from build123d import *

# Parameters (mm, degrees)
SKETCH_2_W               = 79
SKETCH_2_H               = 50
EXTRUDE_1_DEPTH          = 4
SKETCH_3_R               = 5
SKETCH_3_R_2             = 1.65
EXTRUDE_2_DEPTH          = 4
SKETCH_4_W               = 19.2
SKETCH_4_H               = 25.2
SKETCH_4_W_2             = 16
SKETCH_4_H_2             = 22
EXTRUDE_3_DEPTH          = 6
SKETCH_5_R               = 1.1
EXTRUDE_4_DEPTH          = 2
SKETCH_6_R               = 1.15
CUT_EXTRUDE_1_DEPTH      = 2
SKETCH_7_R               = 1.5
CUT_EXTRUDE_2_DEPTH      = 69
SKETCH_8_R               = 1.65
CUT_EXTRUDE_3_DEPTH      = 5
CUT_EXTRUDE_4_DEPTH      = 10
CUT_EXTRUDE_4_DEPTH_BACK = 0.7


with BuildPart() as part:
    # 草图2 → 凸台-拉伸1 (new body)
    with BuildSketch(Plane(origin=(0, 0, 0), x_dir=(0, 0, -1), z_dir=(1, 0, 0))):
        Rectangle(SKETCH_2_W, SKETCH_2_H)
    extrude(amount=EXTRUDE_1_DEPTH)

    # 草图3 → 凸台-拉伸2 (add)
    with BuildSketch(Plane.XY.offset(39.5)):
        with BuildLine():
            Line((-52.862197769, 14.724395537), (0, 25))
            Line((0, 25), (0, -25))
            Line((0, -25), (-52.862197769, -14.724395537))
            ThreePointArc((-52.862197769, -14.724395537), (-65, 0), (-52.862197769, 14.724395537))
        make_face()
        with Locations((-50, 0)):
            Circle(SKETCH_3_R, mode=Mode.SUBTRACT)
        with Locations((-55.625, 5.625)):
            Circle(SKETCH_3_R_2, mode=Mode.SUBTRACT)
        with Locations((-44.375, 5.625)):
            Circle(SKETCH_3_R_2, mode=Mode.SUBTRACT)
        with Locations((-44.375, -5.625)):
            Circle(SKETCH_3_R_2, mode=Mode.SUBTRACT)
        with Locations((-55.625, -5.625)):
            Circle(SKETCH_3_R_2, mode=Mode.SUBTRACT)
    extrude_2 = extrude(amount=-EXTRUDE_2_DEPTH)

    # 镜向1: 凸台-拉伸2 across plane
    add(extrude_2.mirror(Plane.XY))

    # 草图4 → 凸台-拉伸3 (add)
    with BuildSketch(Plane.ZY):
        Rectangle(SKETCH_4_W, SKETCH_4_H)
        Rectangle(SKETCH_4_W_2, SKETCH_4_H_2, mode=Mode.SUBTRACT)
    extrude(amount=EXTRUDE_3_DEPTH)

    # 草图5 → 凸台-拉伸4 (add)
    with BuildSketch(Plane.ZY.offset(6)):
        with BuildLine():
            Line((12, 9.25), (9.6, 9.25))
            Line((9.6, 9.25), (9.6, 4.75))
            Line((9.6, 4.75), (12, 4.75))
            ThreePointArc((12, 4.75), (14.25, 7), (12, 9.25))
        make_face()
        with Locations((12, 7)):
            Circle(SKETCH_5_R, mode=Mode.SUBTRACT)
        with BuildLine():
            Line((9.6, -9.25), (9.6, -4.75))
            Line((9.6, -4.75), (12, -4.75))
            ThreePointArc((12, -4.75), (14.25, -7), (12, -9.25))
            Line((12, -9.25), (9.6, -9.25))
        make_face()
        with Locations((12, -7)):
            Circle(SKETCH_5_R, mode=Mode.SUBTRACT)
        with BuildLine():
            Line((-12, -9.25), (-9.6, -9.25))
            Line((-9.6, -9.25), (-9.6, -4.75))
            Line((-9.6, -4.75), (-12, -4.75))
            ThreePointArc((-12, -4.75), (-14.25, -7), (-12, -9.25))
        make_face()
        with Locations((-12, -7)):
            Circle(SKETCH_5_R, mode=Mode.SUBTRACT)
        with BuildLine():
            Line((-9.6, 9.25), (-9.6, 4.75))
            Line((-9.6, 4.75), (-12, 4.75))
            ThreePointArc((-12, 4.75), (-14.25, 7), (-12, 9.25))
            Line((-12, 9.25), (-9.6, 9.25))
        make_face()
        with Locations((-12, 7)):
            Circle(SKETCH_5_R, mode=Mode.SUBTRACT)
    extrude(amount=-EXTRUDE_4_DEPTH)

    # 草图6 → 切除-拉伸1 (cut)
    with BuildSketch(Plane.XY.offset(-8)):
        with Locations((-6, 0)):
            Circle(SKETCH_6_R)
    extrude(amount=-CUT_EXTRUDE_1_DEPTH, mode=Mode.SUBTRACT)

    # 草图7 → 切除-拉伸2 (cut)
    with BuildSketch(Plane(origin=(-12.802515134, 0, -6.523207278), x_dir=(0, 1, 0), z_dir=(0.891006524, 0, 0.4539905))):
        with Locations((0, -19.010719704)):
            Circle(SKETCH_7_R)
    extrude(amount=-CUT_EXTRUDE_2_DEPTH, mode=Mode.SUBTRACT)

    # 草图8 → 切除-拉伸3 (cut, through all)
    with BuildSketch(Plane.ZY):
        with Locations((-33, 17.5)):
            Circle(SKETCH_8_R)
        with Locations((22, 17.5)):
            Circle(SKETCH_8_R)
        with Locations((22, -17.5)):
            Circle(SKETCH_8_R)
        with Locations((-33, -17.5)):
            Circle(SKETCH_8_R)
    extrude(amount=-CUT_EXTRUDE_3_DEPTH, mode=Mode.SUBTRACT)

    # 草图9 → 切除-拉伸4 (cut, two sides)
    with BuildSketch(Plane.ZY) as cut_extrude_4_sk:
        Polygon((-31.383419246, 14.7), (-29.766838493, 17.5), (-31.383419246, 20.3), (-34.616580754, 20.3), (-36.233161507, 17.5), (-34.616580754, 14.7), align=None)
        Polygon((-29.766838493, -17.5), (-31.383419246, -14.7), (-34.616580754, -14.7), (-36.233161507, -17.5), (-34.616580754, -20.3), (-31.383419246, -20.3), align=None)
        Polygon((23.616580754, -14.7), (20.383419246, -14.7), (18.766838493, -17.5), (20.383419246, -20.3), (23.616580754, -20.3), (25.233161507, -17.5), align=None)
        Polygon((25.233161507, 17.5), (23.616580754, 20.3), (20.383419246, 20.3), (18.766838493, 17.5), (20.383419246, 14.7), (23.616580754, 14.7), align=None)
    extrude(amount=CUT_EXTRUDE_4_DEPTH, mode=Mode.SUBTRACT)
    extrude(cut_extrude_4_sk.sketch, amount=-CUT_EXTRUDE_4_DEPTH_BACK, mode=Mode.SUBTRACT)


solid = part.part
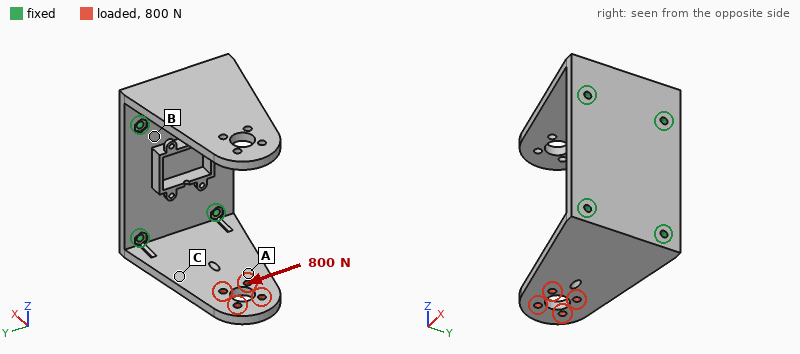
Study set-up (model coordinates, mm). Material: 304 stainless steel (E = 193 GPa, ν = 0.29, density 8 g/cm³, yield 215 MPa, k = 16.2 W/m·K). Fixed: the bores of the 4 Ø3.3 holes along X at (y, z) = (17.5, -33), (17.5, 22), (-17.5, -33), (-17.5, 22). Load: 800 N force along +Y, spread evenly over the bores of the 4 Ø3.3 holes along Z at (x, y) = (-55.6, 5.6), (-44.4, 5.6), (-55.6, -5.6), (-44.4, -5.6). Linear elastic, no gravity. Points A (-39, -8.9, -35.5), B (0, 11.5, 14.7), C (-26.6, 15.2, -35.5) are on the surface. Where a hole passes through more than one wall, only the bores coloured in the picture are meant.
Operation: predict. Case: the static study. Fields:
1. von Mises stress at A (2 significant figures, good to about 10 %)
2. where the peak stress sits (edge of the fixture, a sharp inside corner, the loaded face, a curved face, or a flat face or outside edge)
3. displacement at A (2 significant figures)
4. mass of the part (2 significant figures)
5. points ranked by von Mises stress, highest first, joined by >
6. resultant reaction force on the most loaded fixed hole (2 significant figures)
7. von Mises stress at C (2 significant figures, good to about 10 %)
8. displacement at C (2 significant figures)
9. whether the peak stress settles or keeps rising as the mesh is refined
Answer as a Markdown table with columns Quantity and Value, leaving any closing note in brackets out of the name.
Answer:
| Quantity | Value |
|---|---|
| von Mises stress at A | 9.2 MPa |
| where the peak stress sits | edge of the fixture |
| displacement at A | 17 µm |
| mass of the part | 280 g |
| points ranked by von Mises stress, highest first, joined by > | C > A > B |
| resultant reaction force on the most loaded fixed hole | 1.2 kN |
| von Mises stress at C | 18 MPa |
| displacement at C | 14 µm |
| whether the peak stress settles or keeps rising as the mesh is refined | keeps rising |
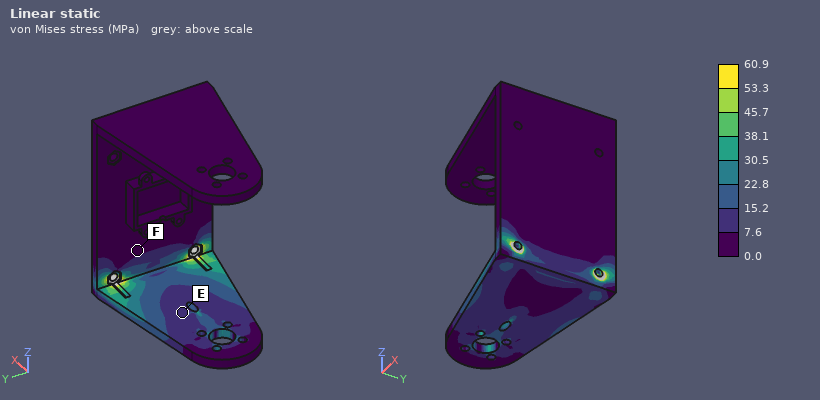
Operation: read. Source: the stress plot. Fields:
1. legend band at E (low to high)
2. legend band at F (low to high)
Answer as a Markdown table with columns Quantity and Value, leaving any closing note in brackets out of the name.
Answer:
| Quantity | Value |
|---|---|
| legend band at E | 7.6 to 15.2 MPa |
| legend band at F | 0.0 to 7.6 MPa |
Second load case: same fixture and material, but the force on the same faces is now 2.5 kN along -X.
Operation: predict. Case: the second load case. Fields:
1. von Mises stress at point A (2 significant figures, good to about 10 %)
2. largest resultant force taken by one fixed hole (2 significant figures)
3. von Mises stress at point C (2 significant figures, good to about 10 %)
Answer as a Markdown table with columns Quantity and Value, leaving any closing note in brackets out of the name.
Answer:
| Quantity | Value |
|---|---|
| von Mises stress at point A | 23 MPa |
| largest resultant force taken by one fixed hole | 1.3 kN |
| von Mises stress at point C | 18 MPa |
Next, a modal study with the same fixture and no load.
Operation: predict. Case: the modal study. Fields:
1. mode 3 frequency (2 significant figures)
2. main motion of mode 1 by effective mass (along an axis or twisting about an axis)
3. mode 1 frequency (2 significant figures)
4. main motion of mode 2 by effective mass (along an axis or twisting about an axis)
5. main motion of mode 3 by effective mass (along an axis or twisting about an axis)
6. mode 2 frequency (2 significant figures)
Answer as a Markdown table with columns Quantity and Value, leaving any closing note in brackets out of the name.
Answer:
| Quantity | Value |
|---|---|
| mode 3 frequency | 2000 Hz |
| main motion of mode 1 by effective mass | along Z |
| mode 1 frequency | 700 Hz |
| main motion of mode 2 by effective mass | along Z |
| main motion of mode 3 by effective mass | along Y |
| mode 2 frequency | 850 Hz |
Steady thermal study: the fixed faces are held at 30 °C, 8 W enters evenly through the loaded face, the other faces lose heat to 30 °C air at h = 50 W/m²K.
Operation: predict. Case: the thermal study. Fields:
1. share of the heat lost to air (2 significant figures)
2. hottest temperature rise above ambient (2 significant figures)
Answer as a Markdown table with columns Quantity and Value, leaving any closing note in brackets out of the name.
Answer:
| Quantity | Value |
|---|---|
| share of the heat lost to air | 88 % |
| hottest temperature rise above ambient | 68 K |
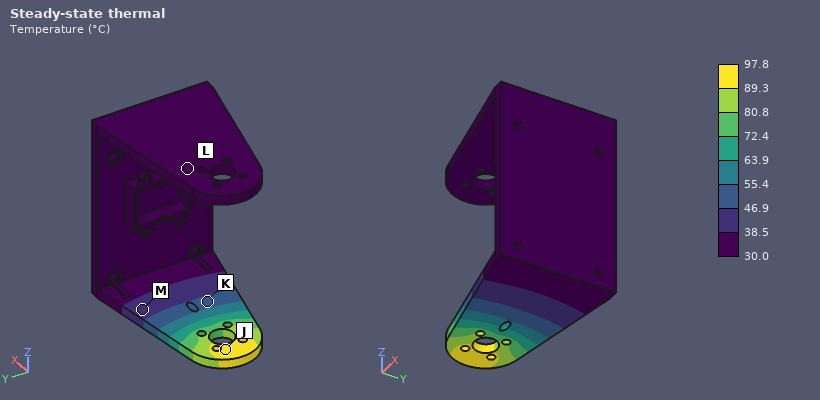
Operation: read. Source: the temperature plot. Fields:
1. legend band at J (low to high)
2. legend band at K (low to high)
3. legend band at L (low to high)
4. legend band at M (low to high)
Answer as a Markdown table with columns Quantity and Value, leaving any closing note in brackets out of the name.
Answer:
| Quantity | Value |
|---|---|
| legend band at J | 89.3 to 97.8 °C |
| legend band at K | 46.9 to 55.4 °C |
| legend band at L | 30.0 to 38.5 °C |
| legend band at M | 38.5 to 46.9 °C |
